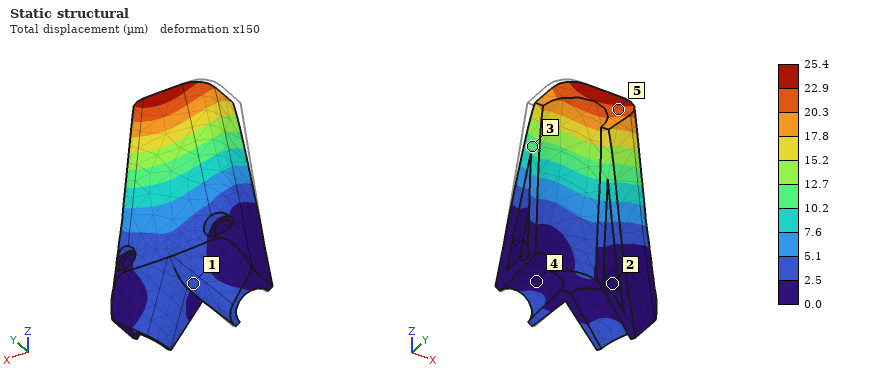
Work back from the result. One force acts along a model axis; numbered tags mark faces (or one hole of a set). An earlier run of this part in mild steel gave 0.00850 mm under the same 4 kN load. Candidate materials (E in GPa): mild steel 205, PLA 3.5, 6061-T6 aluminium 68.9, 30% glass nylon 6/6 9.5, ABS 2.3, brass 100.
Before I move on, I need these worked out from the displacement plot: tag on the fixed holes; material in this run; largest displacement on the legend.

2
6061-T6 aluminium
25.4 µm
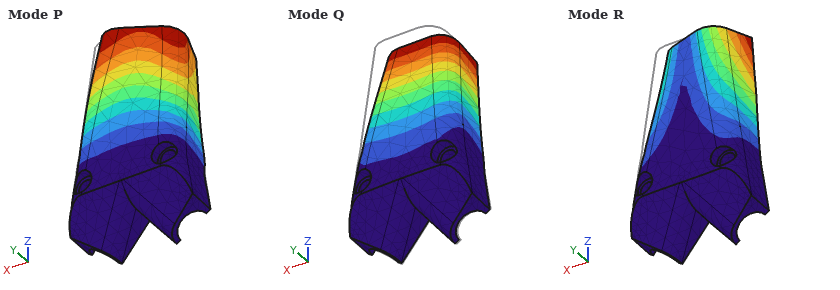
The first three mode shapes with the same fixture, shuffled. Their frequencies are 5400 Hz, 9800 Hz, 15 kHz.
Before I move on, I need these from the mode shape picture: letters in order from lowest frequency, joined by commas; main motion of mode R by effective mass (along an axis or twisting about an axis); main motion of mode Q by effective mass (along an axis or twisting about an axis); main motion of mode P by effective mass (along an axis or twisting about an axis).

Q, R, P
along X
along Y
along X
